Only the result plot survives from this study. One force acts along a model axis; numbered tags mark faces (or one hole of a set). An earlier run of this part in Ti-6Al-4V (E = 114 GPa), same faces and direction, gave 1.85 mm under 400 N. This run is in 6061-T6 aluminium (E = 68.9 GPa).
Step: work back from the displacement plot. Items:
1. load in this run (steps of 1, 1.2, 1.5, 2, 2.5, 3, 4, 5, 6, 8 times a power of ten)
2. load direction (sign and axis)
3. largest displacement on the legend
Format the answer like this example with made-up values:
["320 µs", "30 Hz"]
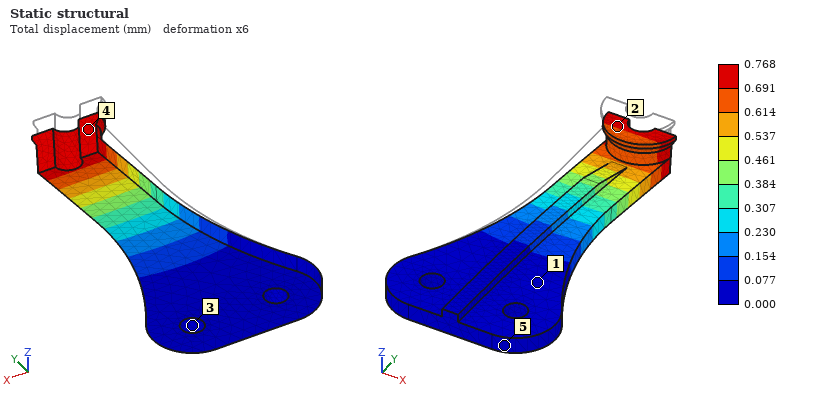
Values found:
["100 N", "-Z", "0.768 mm"]
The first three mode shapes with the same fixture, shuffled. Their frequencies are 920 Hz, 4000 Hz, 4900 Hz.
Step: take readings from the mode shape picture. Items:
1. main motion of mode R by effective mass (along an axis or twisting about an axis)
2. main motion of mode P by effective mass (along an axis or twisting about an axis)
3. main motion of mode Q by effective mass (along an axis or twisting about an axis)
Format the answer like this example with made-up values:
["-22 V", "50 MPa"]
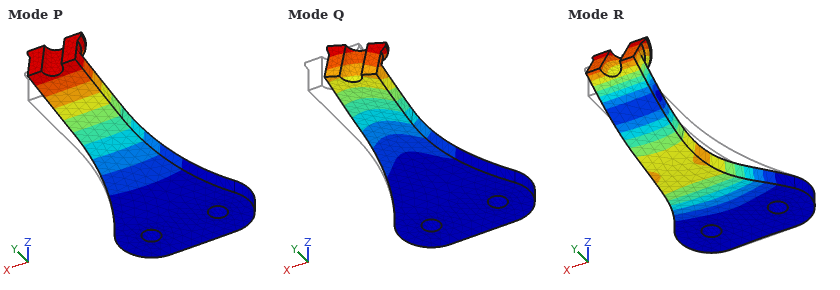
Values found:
["along Z", "along Z", "along X"]
